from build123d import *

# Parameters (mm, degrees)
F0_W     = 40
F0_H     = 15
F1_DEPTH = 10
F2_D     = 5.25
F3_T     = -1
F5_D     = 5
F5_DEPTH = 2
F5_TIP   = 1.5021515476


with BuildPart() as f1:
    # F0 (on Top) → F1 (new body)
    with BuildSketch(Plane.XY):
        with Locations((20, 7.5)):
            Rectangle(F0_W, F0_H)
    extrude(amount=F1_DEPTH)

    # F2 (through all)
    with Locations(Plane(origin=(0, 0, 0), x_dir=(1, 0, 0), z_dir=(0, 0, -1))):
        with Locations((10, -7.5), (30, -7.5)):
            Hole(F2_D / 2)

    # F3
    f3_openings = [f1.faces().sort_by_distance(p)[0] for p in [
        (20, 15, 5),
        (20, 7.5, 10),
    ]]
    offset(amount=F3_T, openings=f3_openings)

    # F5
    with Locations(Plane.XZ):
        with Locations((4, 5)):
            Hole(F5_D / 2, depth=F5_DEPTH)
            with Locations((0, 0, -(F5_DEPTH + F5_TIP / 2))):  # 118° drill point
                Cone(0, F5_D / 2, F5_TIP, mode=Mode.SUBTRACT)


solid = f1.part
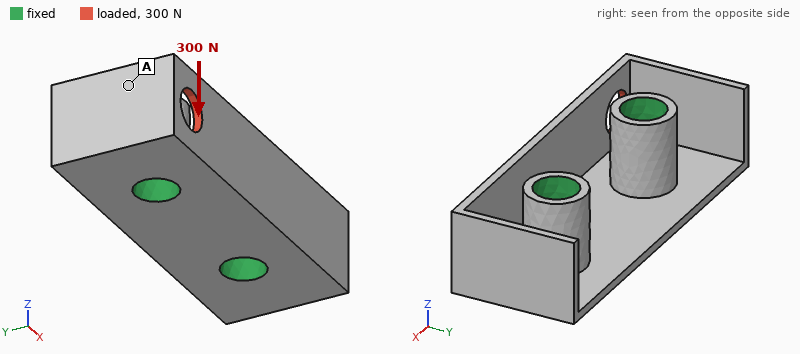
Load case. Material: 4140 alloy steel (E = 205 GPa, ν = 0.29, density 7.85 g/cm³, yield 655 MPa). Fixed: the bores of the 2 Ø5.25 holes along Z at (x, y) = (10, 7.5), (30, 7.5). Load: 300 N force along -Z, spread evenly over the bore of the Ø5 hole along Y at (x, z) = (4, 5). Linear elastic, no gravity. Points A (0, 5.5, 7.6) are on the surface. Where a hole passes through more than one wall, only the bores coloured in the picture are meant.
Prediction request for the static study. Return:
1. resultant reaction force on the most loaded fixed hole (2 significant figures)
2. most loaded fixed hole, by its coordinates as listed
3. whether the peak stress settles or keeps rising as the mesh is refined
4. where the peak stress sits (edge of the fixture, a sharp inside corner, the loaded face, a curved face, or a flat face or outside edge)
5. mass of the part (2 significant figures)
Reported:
360 N
(10, 7.5)
keeps rising
edge of the fixture
12 g
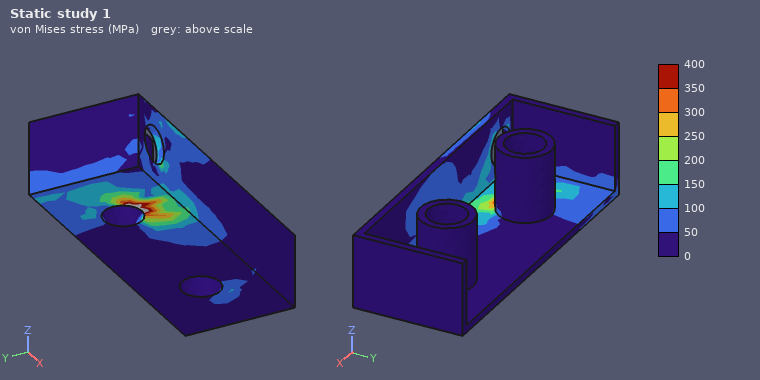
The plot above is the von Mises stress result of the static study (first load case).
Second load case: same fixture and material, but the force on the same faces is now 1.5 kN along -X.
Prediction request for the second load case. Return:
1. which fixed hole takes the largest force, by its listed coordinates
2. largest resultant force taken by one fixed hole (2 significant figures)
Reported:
(10, 7.5)
1000 N
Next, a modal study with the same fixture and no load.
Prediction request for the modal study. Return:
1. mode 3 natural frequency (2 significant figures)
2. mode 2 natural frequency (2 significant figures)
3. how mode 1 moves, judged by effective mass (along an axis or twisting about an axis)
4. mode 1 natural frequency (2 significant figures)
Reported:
7900 Hz
6300 Hz
along Y
5500 Hz
